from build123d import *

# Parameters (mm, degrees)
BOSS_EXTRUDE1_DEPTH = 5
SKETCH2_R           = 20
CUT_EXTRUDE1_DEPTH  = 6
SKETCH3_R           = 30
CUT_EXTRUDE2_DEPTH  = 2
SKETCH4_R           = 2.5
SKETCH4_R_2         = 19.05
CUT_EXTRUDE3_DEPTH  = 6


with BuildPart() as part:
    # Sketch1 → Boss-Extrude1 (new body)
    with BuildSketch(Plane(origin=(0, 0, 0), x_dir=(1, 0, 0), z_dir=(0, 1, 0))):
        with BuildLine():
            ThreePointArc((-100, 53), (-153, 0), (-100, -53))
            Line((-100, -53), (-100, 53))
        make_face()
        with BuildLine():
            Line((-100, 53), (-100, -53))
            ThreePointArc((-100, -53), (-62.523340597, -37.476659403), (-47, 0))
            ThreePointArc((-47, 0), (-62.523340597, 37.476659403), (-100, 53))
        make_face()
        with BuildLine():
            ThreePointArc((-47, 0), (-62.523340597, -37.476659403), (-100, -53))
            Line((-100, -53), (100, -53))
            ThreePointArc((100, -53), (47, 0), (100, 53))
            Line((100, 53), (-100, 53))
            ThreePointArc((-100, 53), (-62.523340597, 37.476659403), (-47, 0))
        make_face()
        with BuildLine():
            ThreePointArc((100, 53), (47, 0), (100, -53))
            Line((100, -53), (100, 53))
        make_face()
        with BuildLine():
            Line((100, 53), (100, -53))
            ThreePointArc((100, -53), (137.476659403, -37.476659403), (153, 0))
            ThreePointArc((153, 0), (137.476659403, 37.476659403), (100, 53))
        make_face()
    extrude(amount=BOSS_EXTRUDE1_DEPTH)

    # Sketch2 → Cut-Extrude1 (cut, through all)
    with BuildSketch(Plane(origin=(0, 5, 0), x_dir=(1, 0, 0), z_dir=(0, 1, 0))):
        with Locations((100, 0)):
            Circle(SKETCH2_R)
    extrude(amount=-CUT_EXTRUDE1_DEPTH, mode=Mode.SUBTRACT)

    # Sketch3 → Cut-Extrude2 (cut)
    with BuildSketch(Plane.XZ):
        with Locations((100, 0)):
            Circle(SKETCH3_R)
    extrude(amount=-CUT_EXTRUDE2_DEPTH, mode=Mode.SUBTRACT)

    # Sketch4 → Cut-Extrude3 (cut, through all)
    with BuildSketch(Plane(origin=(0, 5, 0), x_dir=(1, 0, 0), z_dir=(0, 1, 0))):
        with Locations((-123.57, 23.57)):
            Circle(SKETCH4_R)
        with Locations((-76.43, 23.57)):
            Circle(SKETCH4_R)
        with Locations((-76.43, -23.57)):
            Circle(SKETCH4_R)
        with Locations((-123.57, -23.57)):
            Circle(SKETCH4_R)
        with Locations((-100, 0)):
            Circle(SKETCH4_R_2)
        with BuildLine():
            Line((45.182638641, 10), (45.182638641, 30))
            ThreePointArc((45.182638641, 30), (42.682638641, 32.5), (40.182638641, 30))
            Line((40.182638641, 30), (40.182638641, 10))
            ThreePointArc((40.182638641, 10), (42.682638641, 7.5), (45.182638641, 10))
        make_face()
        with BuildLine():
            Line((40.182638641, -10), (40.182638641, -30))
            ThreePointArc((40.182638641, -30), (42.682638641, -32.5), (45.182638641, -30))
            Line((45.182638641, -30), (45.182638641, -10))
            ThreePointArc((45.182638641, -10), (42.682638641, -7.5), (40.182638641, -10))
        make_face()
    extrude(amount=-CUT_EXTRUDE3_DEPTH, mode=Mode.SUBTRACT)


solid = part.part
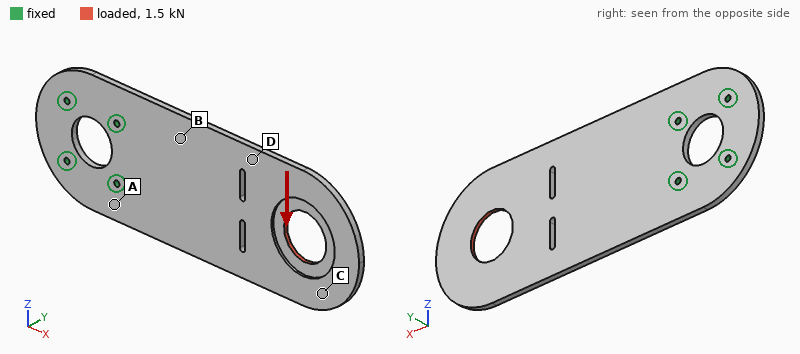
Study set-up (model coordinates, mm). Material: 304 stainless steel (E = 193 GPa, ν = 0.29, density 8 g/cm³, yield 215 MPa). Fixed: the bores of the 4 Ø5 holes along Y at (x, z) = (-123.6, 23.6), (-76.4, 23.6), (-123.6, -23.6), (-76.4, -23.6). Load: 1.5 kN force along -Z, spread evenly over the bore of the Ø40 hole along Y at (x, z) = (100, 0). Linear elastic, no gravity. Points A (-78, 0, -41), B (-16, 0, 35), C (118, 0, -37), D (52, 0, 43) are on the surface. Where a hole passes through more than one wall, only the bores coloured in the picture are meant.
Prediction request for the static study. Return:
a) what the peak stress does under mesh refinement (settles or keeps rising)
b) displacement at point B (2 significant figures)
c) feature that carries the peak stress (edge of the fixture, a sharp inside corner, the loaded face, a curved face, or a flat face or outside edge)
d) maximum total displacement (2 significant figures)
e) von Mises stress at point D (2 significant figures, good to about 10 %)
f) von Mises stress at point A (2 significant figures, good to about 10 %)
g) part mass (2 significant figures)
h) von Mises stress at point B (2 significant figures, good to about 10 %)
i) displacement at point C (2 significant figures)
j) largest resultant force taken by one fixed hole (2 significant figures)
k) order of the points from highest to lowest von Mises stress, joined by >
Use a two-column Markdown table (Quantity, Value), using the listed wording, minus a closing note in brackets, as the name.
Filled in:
| Quantity | Value |
|---|---|
| what the peak stress does under mesh refinement | keeps rising |
| displacement at point B | 16 µm |
| feature that carries the peak stress | edge of the fixture |
| maximum total displacement | 74 µm |
| von Mises stress at point D | 6.1 MPa |
| von Mises stress at point A | 19 MPa |
| part mass | 1.1 kg |
| von Mises stress at point B | 12 MPa |
| displacement at point C | 64 µm |
| largest resultant force taken by one fixed hole | 3.3 kN |
| order of the points from highest to lowest von Mises stress, joined by > | A > B > D > C |
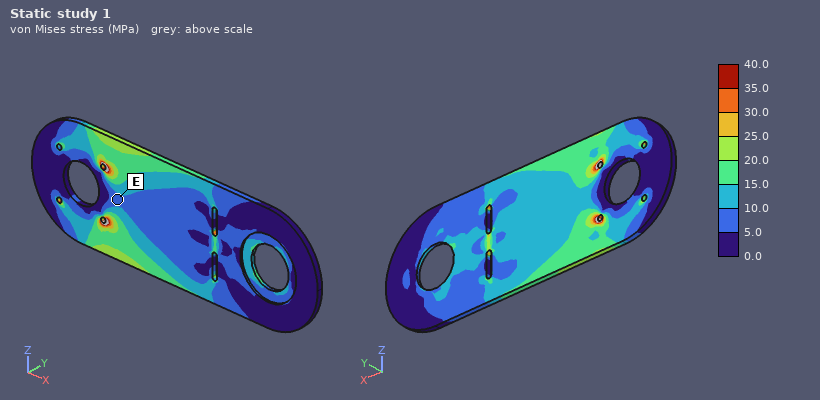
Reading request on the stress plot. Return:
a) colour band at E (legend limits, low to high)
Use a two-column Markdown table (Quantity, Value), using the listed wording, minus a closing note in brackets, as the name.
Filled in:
| Quantity | Value |
|---|---|
| colour band at E | 5.0 to 10.0 MPa |
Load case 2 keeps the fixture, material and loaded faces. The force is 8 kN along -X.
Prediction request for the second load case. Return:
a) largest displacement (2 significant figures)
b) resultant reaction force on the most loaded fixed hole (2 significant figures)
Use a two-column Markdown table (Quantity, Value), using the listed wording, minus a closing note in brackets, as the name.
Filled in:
| Quantity | Value |
|---|---|
| largest displacement | 1.0 mm |
| resultant reaction force on the most loaded fixed hole | 3.4 kN |
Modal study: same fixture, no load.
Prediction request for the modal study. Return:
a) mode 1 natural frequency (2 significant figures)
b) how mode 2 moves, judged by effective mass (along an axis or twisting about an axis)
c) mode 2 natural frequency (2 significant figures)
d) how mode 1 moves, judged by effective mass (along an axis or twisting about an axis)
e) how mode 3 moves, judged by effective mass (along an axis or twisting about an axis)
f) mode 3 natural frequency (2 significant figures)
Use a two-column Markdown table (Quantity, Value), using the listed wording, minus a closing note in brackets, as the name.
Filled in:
| Quantity | Value |
|---|---|
| mode 1 natural frequency | 89 Hz |
| how mode 2 moves, judged by effective mass | twisting about X |
| mode 2 natural frequency | 370 Hz |
| how mode 1 moves, judged by effective mass | along Y |
| how mode 3 moves, judged by effective mass | along Y |
| mode 3 natural frequency | 460 Hz |
